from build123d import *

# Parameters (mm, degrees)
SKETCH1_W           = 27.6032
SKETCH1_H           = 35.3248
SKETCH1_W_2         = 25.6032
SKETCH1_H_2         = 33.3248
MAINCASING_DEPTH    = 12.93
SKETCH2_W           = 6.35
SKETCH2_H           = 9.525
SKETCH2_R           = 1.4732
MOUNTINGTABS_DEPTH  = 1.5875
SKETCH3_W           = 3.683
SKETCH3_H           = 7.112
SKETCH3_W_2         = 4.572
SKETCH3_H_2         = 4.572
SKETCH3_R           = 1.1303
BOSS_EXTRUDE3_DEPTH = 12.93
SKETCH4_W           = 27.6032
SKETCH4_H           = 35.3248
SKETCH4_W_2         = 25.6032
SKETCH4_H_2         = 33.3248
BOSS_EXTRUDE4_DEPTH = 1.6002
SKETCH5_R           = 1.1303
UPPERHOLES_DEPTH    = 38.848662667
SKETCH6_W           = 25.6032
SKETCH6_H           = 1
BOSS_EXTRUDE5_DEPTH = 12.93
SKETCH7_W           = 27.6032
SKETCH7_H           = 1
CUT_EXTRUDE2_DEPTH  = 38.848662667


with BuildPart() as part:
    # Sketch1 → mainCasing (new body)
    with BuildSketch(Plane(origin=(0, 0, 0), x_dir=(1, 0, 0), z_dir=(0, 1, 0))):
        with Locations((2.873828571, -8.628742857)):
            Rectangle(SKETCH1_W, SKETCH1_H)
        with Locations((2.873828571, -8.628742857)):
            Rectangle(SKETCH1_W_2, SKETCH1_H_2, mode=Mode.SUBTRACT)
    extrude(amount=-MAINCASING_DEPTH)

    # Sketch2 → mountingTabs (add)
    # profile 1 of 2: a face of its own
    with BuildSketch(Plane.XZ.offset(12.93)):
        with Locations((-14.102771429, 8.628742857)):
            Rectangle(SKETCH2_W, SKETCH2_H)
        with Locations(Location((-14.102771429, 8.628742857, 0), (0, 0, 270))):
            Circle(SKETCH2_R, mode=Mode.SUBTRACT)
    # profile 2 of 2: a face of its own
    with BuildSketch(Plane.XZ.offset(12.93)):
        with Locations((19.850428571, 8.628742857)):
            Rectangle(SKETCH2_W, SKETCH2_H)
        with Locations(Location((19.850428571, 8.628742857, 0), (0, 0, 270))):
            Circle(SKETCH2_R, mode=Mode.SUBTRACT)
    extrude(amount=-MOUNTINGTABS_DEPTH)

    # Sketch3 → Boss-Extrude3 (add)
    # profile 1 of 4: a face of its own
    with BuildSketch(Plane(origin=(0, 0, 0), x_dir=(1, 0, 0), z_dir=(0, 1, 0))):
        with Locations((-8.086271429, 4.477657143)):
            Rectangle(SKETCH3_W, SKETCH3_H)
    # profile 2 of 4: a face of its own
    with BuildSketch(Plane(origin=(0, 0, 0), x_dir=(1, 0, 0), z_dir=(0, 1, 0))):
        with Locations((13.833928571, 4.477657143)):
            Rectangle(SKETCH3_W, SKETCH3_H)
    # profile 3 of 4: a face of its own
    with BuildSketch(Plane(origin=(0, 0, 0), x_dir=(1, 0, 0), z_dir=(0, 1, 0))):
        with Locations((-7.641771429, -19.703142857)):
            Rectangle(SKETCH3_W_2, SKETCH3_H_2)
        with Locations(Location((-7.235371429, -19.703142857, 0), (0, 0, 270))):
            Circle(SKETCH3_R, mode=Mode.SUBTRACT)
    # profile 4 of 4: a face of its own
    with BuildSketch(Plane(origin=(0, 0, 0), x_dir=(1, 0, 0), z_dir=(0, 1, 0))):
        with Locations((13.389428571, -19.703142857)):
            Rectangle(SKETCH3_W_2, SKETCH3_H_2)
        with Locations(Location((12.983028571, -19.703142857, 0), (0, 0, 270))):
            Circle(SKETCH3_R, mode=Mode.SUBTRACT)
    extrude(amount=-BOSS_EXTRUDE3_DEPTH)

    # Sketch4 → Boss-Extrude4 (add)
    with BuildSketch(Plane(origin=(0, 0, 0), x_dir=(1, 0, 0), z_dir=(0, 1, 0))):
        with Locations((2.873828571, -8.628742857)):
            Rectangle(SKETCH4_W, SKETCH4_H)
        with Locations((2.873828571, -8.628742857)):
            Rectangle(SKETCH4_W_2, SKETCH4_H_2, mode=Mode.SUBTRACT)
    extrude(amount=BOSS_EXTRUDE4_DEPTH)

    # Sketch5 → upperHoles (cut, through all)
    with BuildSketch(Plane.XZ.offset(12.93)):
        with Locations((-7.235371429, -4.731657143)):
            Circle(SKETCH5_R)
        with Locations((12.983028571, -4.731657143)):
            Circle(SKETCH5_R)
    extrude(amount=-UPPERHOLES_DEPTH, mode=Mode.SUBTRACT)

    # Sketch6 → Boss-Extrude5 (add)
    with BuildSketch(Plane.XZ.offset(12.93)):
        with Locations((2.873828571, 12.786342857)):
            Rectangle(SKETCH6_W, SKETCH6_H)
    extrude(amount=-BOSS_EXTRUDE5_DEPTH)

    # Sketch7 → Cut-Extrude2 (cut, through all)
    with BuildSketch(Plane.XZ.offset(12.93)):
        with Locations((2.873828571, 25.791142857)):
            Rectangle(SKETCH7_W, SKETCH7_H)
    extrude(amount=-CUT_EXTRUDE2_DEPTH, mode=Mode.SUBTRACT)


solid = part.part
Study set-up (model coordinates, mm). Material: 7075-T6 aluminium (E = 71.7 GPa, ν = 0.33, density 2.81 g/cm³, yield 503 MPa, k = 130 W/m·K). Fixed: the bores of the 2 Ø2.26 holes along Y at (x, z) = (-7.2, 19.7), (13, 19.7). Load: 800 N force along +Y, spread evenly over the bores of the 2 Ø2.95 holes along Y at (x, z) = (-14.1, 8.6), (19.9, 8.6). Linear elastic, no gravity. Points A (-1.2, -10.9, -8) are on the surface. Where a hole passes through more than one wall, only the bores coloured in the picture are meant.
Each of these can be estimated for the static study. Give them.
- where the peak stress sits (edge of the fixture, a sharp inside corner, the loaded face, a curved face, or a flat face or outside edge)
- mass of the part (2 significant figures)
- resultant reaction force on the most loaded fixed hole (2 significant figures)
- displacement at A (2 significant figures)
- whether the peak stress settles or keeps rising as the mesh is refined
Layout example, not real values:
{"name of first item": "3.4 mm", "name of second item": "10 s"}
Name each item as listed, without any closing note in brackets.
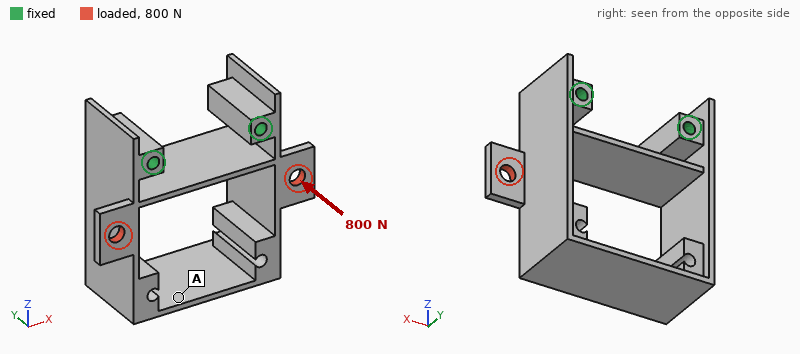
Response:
{"where the peak stress sits": "a sharp inside corner", "mass of the part": "8.1 g", "resultant reaction force on the most loaded fixed hole": "400 N", "displacement at A": "0.053 mm", "whether the peak stress settles or keeps rising as the mesh is refined": "keeps rising"}
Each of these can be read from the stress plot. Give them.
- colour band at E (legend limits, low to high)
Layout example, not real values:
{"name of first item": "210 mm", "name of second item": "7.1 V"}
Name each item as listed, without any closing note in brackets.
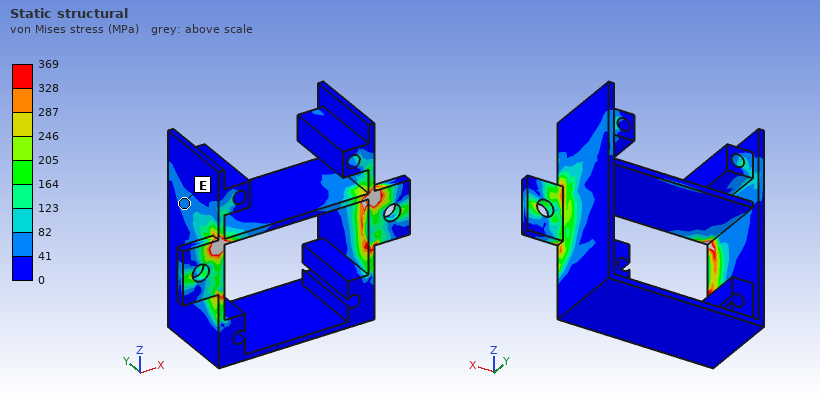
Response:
{"colour band at E": "41 to 82 MPa"}
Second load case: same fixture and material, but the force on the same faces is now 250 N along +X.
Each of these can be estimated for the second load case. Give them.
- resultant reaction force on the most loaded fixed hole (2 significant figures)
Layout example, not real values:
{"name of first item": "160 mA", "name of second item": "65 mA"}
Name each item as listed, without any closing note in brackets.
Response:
{"resultant reaction force on the most loaded fixed hole": "150 N"}
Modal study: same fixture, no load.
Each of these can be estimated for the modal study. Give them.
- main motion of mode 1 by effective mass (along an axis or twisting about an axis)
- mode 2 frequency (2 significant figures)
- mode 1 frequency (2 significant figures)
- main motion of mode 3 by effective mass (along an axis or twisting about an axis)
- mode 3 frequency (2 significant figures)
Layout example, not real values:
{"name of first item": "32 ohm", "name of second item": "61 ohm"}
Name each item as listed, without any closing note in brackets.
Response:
{"main motion of mode 1 by effective mass": "along X", "mode 2 frequency": "5200 Hz", "mode 1 frequency": "1400 Hz", "main motion of mode 3 by effective mass": "along Y", "mode 3 frequency": "5500 Hz"}
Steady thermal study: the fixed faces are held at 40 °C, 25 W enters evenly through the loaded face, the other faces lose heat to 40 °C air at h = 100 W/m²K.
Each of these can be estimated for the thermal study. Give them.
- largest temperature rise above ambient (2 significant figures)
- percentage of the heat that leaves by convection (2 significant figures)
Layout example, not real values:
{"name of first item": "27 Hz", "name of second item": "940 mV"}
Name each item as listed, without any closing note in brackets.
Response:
{"largest temperature rise above ambient": "81 K", "percentage of the heat that leaves by convection": "41 %"}
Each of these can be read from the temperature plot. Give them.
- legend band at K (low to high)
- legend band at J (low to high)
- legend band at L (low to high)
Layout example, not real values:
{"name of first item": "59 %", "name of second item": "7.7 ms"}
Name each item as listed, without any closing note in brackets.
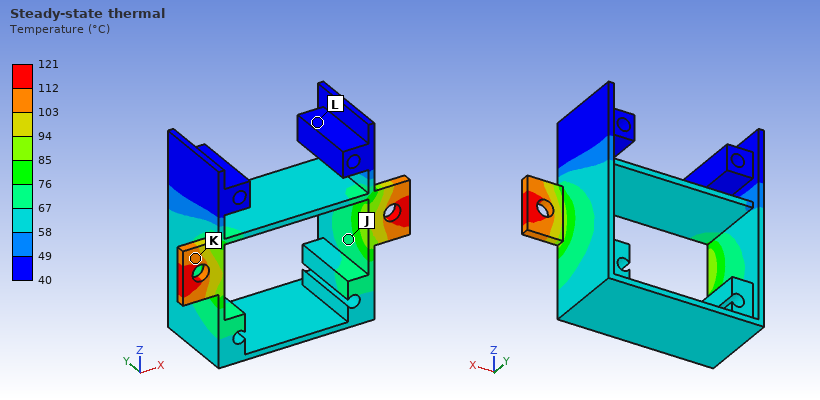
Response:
{"legend band at K": "103 to 112 °C", "legend band at J": "67 to 76 °C", "legend band at L": "40 to 49 °C"}
